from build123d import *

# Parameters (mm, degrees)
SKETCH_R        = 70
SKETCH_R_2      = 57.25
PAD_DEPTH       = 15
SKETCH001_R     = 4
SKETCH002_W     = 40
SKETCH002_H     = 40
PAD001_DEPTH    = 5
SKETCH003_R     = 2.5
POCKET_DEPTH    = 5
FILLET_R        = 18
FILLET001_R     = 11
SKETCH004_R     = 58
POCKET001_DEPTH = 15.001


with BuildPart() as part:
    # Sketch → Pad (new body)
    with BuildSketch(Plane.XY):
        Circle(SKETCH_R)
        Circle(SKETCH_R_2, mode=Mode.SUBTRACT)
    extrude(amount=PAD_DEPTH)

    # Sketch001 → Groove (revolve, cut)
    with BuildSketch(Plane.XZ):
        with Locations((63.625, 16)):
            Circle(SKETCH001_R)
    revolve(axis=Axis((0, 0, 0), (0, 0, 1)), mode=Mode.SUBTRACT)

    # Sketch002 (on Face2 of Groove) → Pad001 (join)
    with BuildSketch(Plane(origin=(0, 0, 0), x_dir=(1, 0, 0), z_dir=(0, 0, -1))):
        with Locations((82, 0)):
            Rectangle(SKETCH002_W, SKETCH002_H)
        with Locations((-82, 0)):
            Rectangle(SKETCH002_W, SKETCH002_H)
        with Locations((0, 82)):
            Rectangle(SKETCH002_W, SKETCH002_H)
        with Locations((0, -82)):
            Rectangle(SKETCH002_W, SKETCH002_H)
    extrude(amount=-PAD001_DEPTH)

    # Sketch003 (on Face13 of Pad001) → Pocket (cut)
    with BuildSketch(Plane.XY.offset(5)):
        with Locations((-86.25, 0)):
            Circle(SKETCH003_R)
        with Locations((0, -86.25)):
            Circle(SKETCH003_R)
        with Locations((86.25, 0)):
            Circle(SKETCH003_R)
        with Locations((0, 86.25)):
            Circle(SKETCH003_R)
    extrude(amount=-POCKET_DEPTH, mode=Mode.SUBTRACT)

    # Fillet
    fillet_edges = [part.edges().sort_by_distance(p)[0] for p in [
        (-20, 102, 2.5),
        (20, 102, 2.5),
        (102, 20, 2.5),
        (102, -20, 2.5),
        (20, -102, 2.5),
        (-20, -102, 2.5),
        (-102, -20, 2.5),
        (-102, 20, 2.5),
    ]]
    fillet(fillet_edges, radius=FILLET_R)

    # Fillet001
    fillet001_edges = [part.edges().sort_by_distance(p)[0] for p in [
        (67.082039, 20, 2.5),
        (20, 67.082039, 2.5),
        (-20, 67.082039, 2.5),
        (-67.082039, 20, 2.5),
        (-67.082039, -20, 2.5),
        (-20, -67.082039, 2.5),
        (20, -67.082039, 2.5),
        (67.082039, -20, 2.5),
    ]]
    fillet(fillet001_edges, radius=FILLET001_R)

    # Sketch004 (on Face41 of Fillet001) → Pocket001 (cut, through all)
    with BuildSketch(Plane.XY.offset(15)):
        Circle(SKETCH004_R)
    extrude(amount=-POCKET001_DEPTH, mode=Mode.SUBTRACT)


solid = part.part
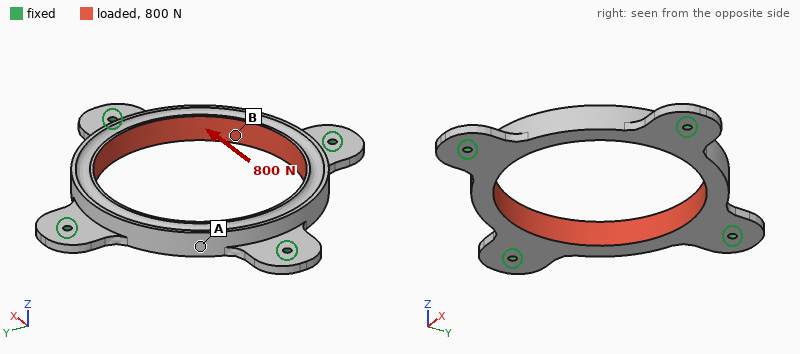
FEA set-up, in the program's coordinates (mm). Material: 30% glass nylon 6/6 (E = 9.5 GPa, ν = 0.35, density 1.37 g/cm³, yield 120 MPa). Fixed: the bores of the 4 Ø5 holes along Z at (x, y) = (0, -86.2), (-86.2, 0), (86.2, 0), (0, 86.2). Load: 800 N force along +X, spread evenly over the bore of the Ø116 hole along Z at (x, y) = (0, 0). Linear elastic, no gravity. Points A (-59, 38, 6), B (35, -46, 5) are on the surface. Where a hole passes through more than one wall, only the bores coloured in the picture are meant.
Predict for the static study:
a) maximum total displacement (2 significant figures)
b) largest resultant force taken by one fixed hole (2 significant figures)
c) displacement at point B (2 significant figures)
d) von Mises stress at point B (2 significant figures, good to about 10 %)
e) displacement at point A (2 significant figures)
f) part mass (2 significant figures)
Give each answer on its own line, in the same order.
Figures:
42 µm
200 N
37 µm
1.9 MPa
25 µm
120 g
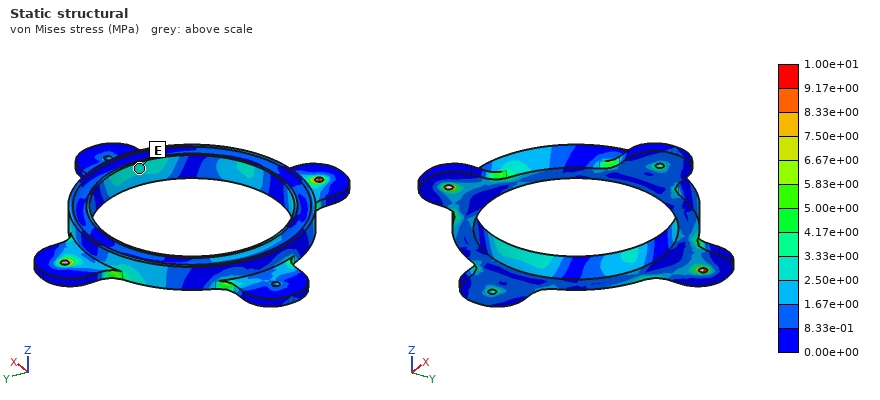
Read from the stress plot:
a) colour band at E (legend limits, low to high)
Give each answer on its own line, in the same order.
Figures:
2.50e+00 to 3.33e+00 MPa
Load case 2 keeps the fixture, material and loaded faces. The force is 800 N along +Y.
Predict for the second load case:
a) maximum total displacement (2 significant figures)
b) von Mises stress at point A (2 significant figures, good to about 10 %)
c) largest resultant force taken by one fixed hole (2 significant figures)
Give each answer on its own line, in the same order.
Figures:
42 µm
2.4 MPa
200 N
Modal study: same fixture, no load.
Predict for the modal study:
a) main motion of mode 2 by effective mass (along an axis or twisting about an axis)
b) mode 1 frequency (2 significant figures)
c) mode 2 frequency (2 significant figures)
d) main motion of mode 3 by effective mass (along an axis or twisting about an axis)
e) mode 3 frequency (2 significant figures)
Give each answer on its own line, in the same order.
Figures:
along Z
1300 Hz
1400 Hz
twisting about Y
1500 Hz
